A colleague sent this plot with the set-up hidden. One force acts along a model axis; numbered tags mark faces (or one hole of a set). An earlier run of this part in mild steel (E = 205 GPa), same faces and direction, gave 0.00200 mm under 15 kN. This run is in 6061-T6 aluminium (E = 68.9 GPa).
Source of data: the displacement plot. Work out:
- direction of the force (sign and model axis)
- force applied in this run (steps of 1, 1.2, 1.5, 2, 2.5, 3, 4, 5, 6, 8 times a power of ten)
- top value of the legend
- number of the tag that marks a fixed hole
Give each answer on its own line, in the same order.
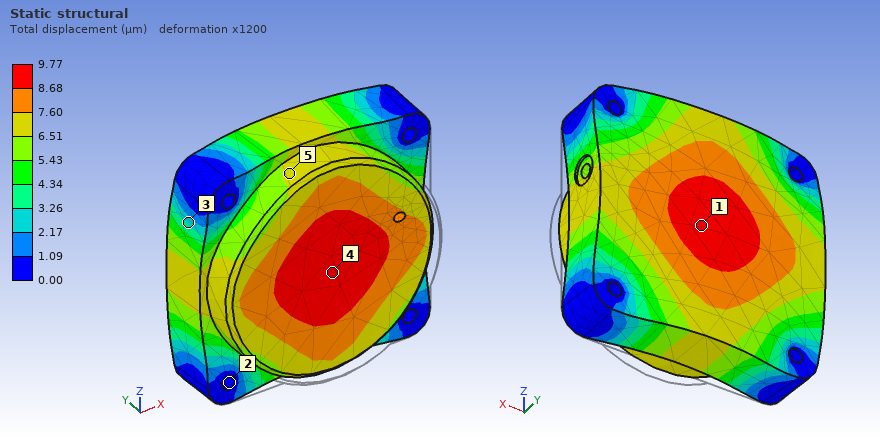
+Y
25 kN
9.77 µm
2
